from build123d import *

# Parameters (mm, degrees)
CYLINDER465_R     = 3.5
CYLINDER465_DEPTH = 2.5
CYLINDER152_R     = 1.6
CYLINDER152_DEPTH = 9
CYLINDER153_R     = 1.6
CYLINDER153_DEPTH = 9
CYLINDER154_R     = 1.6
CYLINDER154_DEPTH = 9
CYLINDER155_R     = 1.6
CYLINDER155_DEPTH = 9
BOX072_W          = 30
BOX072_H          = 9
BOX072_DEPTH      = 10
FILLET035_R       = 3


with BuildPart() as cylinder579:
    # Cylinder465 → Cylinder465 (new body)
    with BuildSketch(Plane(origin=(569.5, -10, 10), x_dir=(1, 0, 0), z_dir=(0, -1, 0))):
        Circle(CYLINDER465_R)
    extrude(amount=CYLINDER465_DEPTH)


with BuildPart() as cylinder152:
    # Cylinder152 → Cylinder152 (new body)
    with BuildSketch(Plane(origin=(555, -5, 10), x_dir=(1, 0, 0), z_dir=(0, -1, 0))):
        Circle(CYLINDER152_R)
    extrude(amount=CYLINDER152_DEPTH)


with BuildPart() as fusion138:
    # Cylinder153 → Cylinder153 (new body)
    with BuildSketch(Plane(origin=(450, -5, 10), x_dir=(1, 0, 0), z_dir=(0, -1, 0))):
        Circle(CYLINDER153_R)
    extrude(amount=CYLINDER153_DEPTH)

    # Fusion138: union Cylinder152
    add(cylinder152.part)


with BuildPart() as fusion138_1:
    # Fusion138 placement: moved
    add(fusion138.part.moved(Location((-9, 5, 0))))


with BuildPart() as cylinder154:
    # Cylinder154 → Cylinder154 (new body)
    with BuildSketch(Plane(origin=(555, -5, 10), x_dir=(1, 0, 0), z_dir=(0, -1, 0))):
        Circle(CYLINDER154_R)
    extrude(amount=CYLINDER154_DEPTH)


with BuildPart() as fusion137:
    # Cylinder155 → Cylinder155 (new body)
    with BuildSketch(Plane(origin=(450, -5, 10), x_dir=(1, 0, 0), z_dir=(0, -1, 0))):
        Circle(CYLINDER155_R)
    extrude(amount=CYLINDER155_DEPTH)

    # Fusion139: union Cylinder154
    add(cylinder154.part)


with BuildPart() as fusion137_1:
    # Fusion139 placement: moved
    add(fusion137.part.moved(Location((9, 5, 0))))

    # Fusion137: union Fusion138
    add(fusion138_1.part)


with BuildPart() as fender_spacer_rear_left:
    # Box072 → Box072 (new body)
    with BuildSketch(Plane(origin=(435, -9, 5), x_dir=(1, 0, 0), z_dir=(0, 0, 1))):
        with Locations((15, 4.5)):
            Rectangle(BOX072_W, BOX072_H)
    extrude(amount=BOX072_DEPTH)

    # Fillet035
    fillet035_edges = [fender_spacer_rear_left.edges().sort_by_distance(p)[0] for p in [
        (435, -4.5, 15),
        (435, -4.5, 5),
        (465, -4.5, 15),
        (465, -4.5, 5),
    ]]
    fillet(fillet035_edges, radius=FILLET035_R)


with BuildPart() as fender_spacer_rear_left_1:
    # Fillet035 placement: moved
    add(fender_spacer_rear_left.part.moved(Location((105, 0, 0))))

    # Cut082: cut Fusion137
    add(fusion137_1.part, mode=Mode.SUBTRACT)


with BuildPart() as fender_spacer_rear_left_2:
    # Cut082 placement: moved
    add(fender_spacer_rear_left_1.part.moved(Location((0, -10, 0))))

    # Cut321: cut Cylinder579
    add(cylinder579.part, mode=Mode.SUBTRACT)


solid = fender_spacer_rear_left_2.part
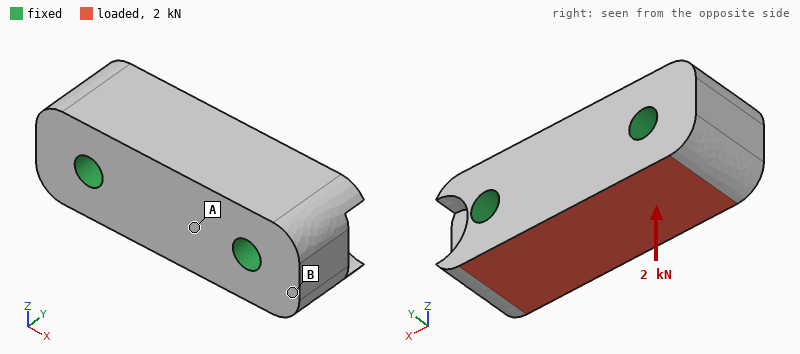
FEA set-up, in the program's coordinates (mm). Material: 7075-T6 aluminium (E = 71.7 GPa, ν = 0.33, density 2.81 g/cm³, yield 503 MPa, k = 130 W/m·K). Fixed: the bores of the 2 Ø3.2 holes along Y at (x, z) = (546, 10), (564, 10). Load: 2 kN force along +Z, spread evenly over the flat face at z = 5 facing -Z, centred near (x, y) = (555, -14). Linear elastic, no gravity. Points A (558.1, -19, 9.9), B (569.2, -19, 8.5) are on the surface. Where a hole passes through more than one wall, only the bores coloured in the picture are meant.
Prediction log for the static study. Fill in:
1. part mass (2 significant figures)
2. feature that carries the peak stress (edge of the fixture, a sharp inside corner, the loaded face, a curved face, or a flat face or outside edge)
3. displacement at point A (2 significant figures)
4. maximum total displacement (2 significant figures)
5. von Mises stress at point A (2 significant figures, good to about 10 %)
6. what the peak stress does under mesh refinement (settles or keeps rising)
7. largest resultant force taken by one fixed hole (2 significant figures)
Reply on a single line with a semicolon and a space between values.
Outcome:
6.8 g; edge of the fixture; 1.8 µm; 2.5 µm; 8.3 MPa; keeps rising; 1.0 kN
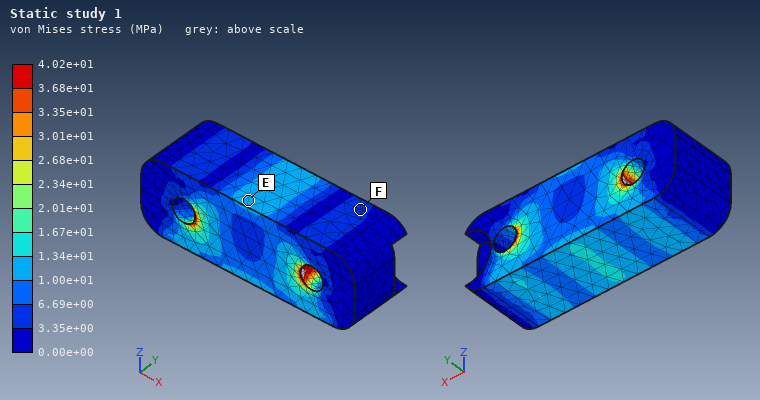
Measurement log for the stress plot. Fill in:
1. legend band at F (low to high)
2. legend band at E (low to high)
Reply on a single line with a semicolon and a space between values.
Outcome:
3.35e+00 to 6.69e+00 MPa; 1.00e+01 to 1.34e+01 MPa
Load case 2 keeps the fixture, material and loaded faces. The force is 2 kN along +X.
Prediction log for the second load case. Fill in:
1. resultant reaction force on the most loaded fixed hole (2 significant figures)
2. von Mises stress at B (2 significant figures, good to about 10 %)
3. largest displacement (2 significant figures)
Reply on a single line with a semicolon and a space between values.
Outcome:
1.1 kN; 5.4 MPa; 2.9 µm
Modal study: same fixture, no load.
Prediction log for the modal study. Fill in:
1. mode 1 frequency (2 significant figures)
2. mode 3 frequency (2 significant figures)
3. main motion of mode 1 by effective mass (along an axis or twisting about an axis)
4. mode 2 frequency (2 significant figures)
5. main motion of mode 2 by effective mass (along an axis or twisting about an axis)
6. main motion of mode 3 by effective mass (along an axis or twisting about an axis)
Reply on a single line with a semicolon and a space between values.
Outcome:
66 kHz; 80 kHz; along Z; 72 kHz; along Y; twisting about X
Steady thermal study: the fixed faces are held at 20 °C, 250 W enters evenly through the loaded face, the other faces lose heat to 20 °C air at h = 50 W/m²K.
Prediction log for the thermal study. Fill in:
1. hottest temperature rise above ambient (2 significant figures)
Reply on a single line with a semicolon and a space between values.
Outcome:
66 K
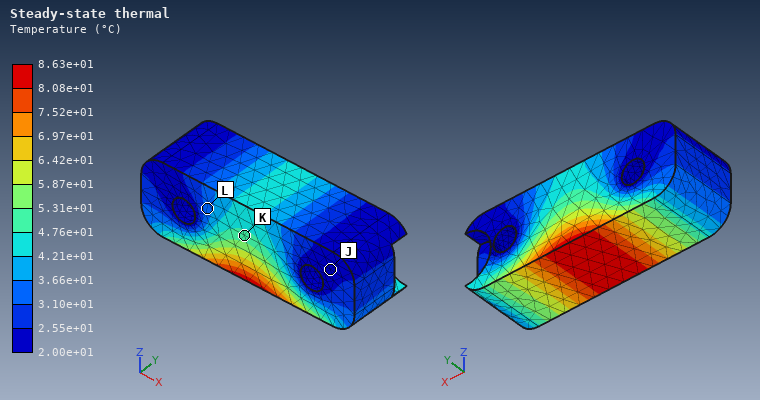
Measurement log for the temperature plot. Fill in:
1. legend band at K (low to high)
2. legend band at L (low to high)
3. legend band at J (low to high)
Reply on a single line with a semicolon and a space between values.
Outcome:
4.76e+01 to 5.31e+01 °C; 3.10e+01 to 3.66e+01 °C; 2.00e+01 to 2.55e+01 °C
